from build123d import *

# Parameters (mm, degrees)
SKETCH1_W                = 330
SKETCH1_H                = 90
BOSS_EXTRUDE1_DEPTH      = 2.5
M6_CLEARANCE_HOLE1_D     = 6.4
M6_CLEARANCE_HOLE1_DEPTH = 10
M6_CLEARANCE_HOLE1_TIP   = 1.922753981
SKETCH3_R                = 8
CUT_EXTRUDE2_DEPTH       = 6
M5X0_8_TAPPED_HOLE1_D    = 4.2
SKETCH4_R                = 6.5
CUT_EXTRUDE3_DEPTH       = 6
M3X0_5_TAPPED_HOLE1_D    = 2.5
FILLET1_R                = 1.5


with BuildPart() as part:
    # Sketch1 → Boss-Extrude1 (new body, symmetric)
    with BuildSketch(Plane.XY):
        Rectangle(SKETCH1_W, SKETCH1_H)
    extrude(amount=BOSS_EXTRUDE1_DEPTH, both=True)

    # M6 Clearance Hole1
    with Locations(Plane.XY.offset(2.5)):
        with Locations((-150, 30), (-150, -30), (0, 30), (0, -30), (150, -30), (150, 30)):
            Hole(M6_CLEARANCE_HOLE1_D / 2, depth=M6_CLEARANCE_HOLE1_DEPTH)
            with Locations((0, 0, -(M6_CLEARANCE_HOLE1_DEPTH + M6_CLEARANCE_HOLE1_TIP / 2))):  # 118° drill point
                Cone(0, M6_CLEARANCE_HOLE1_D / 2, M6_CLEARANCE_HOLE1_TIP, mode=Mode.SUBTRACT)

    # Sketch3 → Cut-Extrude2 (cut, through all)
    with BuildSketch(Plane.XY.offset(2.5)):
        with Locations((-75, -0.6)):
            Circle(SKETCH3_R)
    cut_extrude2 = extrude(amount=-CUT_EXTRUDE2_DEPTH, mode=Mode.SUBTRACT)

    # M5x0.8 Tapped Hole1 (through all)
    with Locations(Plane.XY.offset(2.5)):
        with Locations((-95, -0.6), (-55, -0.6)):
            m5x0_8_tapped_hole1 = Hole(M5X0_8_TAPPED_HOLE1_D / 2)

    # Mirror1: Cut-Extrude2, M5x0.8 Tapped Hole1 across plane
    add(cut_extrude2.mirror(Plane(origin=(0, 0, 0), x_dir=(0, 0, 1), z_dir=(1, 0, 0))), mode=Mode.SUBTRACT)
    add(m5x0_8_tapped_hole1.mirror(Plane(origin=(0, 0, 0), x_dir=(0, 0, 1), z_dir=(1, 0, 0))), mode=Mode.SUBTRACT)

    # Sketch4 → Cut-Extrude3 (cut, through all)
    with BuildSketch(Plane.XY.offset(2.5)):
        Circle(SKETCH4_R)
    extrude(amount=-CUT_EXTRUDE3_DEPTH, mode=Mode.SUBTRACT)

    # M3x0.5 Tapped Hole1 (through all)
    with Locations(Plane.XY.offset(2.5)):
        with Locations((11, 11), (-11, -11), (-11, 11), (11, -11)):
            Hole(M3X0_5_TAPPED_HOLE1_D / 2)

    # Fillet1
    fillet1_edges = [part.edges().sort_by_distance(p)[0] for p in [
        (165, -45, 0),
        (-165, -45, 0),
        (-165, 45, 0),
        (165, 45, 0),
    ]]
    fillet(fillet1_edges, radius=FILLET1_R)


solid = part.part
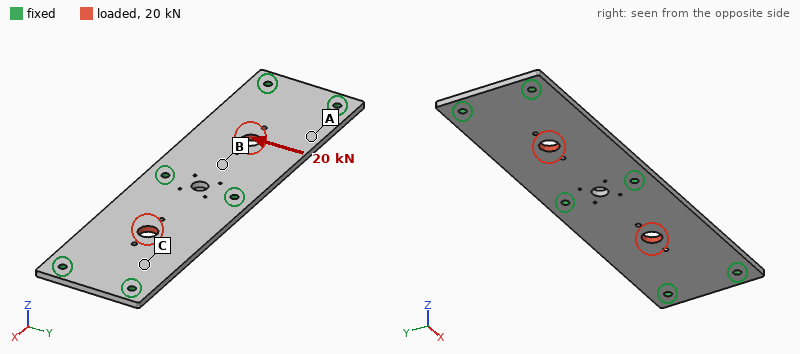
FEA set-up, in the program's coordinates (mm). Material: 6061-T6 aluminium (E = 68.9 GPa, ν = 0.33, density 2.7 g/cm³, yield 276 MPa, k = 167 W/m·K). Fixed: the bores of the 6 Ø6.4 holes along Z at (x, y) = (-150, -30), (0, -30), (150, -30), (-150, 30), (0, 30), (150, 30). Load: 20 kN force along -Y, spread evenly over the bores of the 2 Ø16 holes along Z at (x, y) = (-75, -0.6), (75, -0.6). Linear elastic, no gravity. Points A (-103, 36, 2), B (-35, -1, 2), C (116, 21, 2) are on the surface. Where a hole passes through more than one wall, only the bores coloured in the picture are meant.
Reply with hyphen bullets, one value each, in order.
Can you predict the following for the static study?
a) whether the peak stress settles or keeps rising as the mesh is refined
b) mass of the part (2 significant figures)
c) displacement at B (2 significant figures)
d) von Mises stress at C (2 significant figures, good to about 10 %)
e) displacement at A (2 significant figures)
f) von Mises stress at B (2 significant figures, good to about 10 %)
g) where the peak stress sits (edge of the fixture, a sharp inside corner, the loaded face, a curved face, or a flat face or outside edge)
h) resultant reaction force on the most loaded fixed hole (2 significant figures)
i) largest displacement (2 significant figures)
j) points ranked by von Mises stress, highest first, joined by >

- keeps rising
- 390 g
- 25 µm
- 23 MPa
- 34 µm
- 29 MPa
- edge of the fixture
- 5.2 kN
- 52 µm
- B > C > A
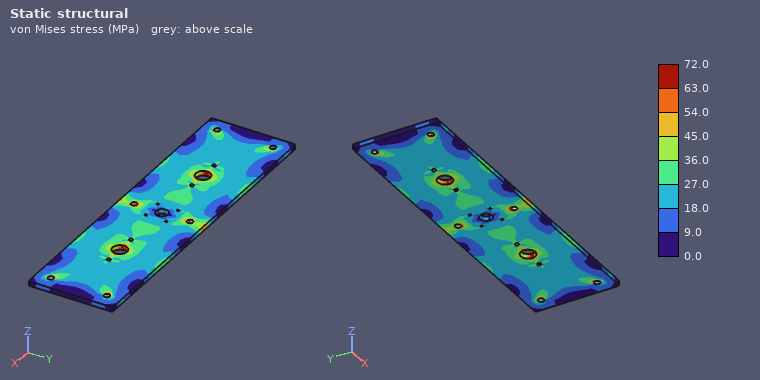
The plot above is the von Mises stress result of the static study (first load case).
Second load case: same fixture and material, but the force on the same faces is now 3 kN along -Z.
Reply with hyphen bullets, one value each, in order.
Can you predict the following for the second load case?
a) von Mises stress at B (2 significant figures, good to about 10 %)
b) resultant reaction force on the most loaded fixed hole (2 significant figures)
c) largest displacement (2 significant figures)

- 19 MPa
- 780 N
- 0.50 mm
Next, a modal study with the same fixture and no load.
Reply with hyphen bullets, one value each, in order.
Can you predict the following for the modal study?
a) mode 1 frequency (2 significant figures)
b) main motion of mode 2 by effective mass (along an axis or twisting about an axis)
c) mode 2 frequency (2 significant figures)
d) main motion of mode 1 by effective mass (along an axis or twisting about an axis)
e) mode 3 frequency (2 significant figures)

- 1100 Hz
- along Z
- 1100 Hz
- twisting about Y
- 1700 Hz
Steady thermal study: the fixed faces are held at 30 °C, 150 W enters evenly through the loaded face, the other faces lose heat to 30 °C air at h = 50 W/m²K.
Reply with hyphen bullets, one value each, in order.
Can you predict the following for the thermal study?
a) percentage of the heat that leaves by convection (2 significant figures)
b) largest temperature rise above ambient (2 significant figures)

- 32 %
- 42 K
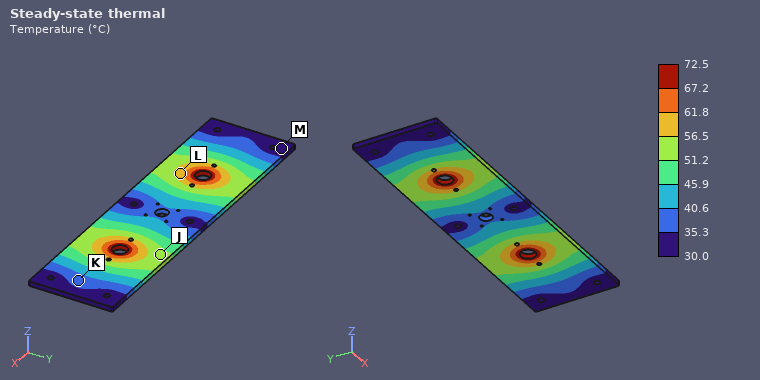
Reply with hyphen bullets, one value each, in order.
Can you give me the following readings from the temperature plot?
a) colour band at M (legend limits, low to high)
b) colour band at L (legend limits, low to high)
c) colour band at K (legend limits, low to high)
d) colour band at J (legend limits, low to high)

- 30.0 to 35.3 °C
- 56.5 to 61.8 °C
- 35.3 to 40.6 °C
- 51.2 to 56.5 °C
